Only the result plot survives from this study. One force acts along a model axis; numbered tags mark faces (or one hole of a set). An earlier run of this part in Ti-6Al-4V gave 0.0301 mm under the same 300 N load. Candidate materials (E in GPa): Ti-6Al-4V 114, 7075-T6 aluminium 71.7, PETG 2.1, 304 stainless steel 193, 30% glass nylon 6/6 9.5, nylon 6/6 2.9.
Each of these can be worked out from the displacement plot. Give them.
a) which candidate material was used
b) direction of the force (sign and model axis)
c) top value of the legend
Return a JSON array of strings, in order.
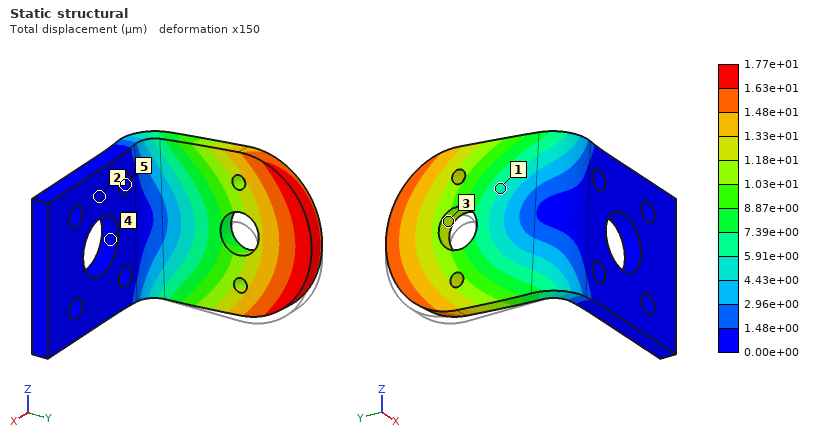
["304 stainless steel", "+Z", "1.77e+01 µm"]
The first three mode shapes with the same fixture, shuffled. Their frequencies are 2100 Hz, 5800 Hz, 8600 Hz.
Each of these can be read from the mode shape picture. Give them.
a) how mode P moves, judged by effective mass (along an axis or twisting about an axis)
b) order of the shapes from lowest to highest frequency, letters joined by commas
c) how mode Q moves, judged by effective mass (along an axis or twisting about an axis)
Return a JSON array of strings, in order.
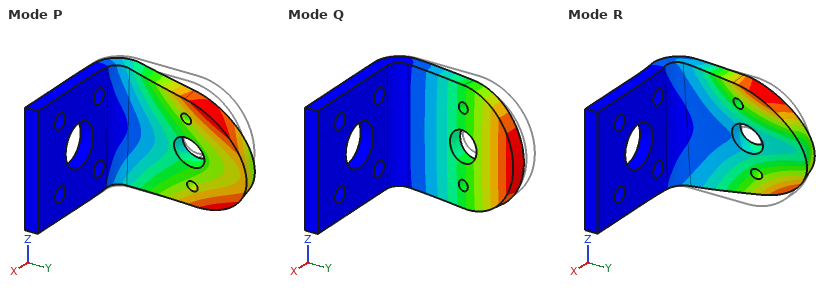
["along Z", "Q, P, R", "along X"]
